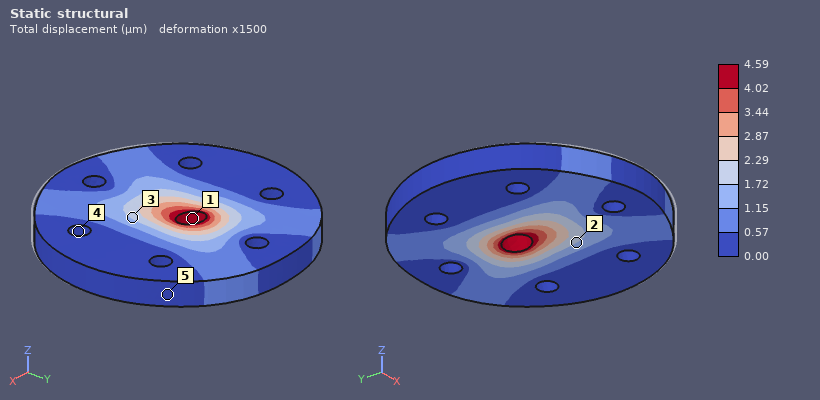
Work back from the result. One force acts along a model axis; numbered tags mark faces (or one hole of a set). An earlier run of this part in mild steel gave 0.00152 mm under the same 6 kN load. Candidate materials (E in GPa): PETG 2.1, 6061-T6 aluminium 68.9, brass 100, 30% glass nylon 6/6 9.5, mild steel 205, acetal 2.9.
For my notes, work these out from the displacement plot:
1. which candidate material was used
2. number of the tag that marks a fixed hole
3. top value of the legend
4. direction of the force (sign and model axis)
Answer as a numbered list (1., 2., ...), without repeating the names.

1. 6061-T6 aluminium
2. 4
3. 4.59 µm
4. +Y
